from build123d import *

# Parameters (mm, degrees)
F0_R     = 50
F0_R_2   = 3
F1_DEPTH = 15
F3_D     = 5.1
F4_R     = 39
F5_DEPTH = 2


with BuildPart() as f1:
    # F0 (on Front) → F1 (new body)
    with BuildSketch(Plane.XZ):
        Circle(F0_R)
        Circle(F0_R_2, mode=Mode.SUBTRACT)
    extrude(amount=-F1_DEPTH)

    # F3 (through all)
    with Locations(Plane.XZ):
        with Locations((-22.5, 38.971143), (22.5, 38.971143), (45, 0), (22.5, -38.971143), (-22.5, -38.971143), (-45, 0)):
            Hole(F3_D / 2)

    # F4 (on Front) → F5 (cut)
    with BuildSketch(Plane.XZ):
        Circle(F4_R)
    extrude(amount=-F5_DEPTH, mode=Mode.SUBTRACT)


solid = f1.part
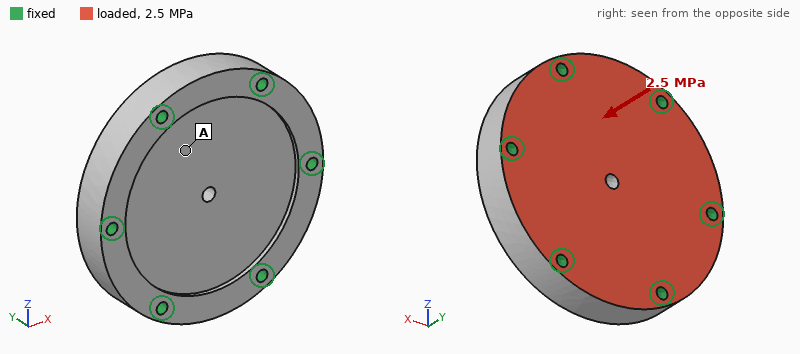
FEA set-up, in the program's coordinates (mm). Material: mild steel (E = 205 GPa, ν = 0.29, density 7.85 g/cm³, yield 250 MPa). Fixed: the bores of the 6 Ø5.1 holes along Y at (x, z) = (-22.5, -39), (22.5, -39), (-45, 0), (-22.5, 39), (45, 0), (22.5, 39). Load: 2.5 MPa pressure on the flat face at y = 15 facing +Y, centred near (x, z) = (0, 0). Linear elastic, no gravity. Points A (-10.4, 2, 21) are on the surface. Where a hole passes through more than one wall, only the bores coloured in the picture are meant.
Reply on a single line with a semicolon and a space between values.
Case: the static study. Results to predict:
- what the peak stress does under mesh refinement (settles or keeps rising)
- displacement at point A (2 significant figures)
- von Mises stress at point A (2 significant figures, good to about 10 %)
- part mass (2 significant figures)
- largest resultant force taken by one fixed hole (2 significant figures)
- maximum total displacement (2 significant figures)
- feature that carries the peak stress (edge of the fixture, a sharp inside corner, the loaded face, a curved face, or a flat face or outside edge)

keeps rising; 4.8 µm; 8.8 MPa; 830 g; 3.2 kN; 7.6 µm; edge of the fixture
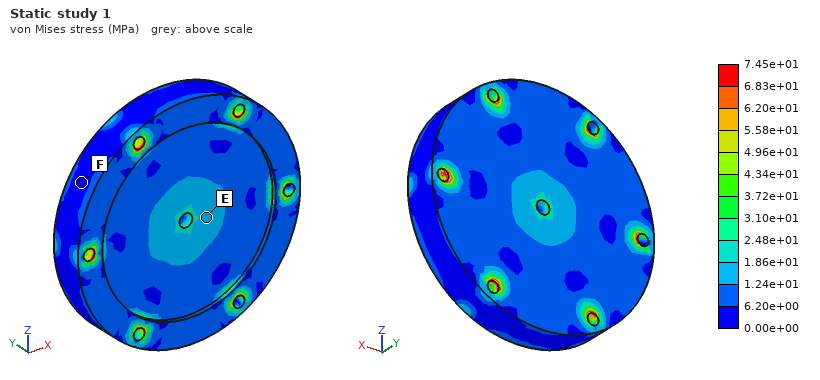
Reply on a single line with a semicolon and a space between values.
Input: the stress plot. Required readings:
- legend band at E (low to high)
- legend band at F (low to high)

1.24e+01 to 1.86e+01 MPa; 0.00e+00 to 6.20e+00 MPa
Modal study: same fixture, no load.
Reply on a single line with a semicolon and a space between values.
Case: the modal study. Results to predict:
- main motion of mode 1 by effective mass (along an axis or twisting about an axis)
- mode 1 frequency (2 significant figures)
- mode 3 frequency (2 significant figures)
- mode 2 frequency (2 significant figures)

along Y; 11 kHz; 20 kHz; 20 kHz
